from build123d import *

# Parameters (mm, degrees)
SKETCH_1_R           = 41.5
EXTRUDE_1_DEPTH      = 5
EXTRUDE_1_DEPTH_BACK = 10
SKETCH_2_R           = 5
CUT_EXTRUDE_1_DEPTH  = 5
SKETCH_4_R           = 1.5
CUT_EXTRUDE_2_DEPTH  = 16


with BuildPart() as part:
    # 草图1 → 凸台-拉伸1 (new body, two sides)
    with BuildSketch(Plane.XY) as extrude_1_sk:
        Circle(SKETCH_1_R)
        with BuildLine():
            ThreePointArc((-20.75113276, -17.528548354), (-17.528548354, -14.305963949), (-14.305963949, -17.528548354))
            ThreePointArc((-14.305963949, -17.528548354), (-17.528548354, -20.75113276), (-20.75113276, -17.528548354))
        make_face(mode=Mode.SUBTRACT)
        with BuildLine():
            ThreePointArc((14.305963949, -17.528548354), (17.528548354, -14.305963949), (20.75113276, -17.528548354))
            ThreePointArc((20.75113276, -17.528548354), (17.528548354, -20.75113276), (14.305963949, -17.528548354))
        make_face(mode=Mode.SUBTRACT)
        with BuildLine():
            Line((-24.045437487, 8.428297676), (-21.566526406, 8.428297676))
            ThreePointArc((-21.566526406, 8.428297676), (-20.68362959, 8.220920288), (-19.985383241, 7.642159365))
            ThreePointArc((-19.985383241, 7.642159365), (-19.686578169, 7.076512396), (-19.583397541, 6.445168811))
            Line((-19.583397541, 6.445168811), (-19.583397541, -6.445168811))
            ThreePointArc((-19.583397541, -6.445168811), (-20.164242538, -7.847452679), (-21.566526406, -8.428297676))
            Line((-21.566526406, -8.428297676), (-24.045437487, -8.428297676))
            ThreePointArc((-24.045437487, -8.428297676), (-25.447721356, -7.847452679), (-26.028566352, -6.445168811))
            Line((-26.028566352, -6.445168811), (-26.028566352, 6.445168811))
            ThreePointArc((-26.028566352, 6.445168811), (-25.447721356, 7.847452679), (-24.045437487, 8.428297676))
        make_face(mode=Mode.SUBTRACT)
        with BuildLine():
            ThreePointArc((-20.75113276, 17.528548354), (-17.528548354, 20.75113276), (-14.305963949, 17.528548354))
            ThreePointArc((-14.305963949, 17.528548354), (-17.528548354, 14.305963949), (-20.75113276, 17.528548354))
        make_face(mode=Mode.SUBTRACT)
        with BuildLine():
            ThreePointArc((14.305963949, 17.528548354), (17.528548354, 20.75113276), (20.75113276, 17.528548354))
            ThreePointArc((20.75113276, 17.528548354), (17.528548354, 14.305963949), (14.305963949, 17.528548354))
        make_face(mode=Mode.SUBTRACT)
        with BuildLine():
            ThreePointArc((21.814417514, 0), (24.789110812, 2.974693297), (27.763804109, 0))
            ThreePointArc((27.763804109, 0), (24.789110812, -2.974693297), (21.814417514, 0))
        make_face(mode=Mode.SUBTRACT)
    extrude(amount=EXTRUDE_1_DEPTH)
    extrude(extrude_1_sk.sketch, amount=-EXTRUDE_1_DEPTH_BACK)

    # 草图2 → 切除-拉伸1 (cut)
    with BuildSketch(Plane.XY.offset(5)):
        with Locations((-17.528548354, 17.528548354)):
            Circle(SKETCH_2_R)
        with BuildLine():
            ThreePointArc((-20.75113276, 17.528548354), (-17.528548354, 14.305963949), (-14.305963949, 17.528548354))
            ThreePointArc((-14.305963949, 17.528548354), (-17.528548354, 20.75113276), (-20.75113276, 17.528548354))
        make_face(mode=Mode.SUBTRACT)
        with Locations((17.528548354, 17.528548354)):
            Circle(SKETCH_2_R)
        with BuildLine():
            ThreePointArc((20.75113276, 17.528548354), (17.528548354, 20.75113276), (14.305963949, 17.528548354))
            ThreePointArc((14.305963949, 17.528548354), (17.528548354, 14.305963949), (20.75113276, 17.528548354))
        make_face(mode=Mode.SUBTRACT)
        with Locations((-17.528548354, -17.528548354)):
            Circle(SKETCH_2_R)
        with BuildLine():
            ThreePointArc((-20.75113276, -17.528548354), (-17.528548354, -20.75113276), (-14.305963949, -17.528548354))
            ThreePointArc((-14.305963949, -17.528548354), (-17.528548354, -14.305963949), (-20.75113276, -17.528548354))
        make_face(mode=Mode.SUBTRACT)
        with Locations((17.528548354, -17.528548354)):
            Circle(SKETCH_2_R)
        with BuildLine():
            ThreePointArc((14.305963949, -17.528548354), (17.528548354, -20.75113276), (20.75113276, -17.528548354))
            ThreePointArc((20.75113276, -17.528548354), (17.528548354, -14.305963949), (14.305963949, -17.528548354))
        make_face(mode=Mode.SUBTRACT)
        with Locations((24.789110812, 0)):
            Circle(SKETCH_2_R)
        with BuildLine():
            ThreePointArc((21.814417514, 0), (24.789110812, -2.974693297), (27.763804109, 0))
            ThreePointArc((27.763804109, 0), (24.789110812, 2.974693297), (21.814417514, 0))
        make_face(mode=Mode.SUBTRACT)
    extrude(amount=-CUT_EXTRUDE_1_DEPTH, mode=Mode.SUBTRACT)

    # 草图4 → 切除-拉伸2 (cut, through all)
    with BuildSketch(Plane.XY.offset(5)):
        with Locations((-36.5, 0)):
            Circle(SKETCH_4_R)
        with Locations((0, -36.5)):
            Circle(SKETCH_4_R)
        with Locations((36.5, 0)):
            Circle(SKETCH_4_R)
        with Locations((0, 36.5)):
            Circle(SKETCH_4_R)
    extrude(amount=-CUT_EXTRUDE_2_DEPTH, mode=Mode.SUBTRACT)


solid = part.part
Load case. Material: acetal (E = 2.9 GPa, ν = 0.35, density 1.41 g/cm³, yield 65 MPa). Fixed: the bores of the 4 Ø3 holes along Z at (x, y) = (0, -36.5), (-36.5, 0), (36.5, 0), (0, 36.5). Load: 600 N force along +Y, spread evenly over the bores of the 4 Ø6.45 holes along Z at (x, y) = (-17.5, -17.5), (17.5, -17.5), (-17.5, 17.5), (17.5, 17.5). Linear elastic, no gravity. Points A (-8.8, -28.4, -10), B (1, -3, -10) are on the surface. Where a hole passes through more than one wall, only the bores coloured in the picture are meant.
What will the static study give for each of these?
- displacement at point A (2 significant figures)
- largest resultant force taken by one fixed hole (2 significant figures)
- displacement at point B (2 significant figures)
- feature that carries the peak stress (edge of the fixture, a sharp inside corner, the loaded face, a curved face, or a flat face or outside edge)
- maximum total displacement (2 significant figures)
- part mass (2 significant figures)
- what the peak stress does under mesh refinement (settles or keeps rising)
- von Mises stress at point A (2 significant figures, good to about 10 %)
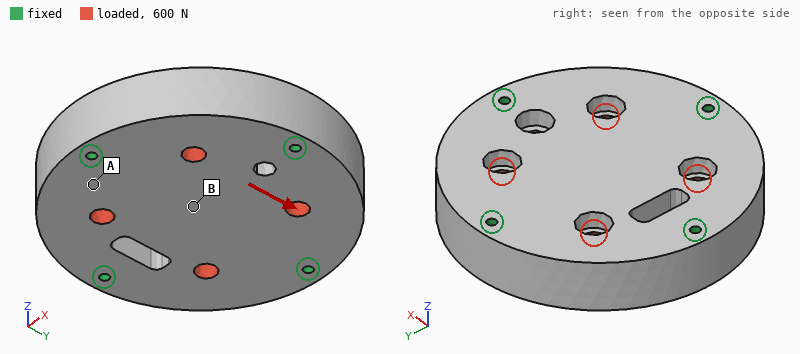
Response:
4.0 µm
170 N
5.1 µm
edge of the fixture
7.6 µm
110 g
keeps rising
0.60 MPa
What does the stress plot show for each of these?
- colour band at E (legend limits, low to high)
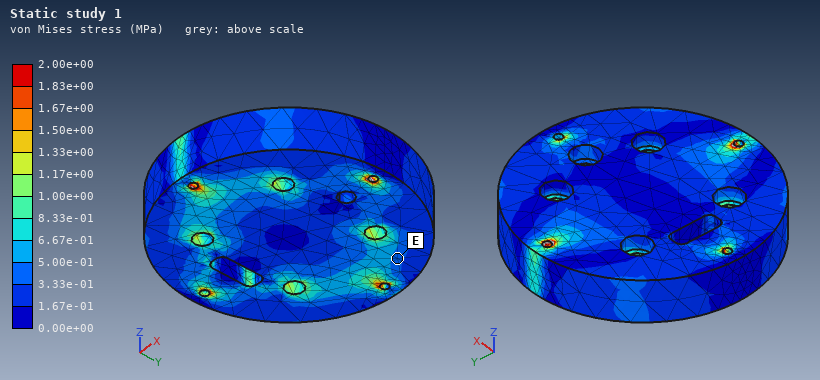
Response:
3.33e-01 to 5.00e-01 MPa
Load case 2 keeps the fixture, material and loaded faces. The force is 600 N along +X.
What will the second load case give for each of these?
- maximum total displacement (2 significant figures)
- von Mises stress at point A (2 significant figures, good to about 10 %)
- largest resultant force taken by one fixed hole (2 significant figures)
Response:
8.3 µm
0.45 MPa
160 N
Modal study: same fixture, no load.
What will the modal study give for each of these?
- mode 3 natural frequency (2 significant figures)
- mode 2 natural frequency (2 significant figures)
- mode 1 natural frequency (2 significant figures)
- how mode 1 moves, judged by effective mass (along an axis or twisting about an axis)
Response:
4400 Hz
4300 Hz
3500 Hz
along Z
